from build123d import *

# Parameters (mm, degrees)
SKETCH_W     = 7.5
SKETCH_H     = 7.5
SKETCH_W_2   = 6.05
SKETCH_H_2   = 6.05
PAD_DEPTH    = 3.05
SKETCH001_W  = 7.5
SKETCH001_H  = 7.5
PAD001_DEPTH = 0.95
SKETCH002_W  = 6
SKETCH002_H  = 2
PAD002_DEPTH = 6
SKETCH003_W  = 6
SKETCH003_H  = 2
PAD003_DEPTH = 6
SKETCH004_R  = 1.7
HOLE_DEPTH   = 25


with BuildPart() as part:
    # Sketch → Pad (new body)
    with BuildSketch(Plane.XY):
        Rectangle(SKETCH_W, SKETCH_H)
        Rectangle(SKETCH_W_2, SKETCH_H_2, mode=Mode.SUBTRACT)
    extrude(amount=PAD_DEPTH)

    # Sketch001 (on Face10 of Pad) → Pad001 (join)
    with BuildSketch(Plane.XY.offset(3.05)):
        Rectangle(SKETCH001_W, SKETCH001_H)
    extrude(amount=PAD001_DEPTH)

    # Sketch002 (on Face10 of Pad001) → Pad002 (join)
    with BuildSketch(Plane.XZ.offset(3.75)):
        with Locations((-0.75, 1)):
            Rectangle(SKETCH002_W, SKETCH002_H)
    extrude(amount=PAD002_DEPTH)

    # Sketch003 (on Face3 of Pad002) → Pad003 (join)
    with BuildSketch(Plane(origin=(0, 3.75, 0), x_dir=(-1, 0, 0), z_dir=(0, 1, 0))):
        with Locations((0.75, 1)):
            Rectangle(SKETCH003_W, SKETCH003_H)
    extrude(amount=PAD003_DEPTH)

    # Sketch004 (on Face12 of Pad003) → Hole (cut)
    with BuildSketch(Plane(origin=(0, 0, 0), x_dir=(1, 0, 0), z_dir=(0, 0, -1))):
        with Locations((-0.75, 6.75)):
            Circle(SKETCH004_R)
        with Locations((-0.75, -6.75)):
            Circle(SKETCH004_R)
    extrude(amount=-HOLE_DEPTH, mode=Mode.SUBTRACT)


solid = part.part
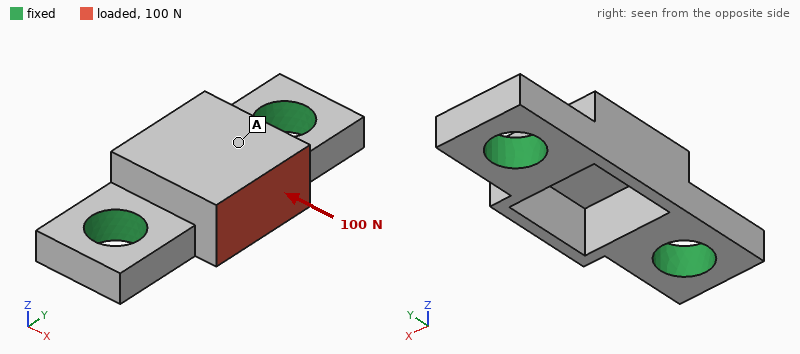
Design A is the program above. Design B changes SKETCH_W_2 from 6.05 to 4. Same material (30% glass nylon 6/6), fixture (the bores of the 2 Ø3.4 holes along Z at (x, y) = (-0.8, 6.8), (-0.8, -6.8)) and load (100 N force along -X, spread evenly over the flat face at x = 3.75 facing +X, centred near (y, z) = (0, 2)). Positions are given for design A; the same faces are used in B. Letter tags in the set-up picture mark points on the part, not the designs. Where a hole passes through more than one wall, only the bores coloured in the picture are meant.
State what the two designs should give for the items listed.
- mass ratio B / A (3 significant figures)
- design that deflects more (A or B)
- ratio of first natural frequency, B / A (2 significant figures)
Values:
1.17
A
0.92
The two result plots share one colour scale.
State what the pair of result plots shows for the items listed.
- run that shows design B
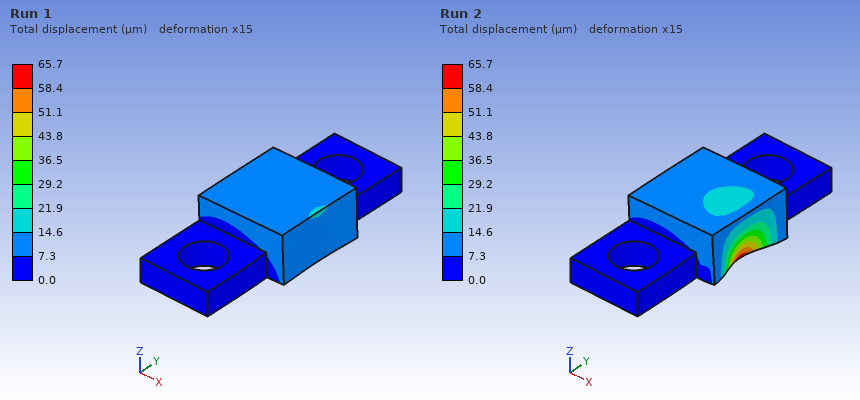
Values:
Run 1
